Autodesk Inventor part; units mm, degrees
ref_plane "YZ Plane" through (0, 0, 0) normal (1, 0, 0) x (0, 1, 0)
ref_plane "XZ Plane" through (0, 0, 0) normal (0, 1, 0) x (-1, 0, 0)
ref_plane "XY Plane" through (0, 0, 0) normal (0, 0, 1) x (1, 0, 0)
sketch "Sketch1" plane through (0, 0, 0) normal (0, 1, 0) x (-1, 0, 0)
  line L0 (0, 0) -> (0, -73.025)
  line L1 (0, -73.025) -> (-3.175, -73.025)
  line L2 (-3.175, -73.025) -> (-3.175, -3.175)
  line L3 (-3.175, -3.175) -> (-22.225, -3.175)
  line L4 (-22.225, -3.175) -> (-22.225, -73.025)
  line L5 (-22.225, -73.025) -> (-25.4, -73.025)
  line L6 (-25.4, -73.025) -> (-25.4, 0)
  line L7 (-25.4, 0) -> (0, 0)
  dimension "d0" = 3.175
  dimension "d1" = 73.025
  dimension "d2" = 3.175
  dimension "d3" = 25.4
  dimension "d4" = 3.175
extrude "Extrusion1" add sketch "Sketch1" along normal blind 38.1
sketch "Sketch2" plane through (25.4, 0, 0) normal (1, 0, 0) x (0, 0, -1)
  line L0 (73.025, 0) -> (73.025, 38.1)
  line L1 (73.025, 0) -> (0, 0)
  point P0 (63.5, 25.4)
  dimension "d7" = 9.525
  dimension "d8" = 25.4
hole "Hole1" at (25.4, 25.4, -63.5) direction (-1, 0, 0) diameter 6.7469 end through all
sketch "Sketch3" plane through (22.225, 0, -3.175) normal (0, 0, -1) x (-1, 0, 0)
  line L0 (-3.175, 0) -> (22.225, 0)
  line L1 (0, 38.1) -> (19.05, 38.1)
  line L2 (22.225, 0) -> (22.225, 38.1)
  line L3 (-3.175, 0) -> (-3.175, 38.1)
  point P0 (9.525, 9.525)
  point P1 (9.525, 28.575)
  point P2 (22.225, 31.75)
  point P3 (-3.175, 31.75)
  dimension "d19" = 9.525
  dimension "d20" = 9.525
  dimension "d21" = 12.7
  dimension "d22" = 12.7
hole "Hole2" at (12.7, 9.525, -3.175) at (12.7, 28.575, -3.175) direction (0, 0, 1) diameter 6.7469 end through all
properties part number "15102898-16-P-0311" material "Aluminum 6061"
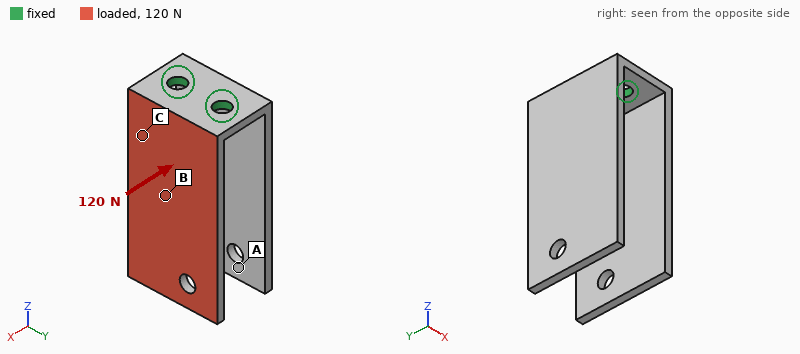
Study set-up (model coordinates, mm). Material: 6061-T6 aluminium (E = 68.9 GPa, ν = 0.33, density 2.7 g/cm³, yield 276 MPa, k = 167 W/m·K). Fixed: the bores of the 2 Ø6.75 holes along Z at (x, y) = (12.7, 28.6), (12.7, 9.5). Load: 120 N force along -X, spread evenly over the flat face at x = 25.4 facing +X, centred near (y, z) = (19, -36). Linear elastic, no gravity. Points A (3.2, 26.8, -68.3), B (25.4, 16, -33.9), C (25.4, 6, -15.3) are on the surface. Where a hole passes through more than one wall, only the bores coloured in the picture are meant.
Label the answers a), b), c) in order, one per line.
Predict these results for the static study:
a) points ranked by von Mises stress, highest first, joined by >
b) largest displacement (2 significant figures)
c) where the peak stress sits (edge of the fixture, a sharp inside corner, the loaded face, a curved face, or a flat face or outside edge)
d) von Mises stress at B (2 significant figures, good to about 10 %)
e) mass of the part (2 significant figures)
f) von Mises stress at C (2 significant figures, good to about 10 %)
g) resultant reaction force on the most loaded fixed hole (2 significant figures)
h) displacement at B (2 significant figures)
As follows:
a) C > B > A
b) 1.0 mm
c) a flat face or outside edge
d) 18 MPa
e) 53 g
f) 41 MPa
g) 67 N
h) 0.36 mm
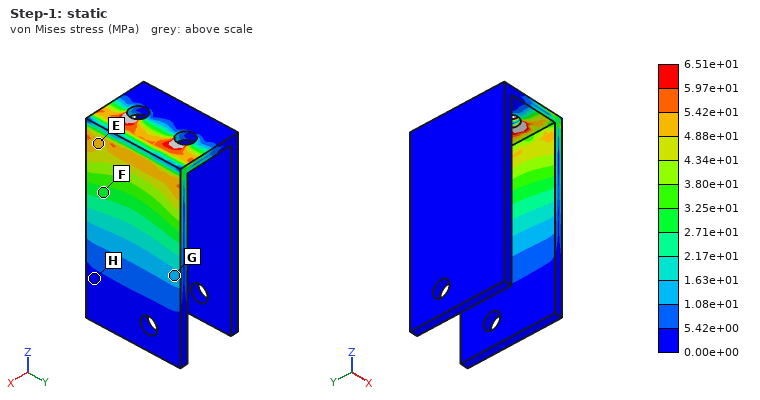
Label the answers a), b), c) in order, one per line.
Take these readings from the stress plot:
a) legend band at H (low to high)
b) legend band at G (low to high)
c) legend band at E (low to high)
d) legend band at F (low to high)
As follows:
a) 0.00e+00 to 5.42e+00 MPa
b) 1.08e+01 to 1.63e+01 MPa
c) 4.88e+01 to 5.42e+01 MPa
d) 2.71e+01 to 3.25e+01 MPa
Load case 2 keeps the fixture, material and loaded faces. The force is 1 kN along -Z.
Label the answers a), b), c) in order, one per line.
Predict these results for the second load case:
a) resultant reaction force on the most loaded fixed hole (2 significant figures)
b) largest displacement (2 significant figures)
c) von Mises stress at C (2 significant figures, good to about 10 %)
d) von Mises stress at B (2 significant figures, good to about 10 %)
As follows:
a) 500 N
b) 0.89 mm
c) 26 MPa
d) 17 MPa
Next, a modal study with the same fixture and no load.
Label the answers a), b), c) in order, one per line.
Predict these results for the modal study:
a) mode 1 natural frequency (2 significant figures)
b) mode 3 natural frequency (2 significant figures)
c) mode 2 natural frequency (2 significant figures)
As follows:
a) 440 Hz
b) 1600 Hz
c) 440 Hz
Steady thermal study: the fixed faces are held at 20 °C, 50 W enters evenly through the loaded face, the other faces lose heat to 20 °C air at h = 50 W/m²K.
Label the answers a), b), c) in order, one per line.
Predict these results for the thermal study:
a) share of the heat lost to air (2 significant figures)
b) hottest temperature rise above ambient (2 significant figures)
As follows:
a) 22 %
b) 81 K
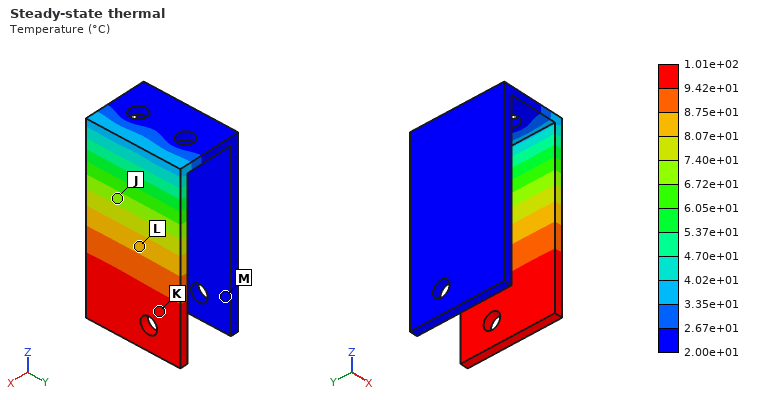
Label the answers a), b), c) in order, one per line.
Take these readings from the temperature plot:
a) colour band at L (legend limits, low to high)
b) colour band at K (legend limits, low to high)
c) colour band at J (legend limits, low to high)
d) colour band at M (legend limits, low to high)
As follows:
a) 8.07e+01 to 8.75e+01 °C
b) 9.42e+01 to 1.01e+02 °C
c) 6.72e+01 to 7.40e+01 °C
d) 2.00e+01 to 2.67e+01 °C
